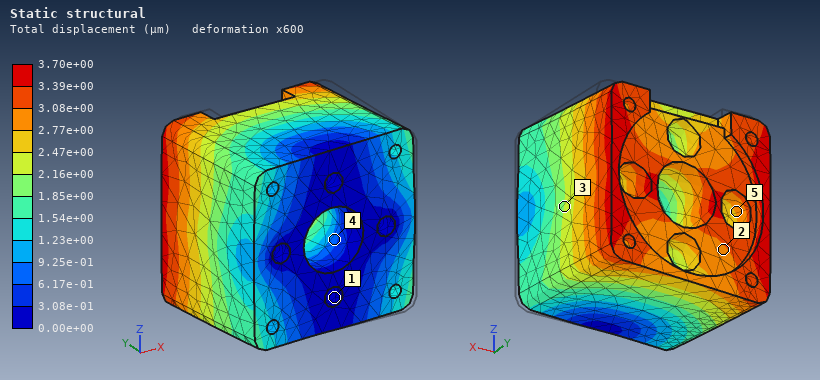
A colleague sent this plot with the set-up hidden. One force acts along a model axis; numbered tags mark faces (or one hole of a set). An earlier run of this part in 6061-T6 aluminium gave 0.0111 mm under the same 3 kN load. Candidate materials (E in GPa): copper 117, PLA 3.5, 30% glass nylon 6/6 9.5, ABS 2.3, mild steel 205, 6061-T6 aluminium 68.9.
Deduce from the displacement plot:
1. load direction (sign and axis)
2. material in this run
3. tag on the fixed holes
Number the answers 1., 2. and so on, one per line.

1. -X
2. mild steel
3. 1
